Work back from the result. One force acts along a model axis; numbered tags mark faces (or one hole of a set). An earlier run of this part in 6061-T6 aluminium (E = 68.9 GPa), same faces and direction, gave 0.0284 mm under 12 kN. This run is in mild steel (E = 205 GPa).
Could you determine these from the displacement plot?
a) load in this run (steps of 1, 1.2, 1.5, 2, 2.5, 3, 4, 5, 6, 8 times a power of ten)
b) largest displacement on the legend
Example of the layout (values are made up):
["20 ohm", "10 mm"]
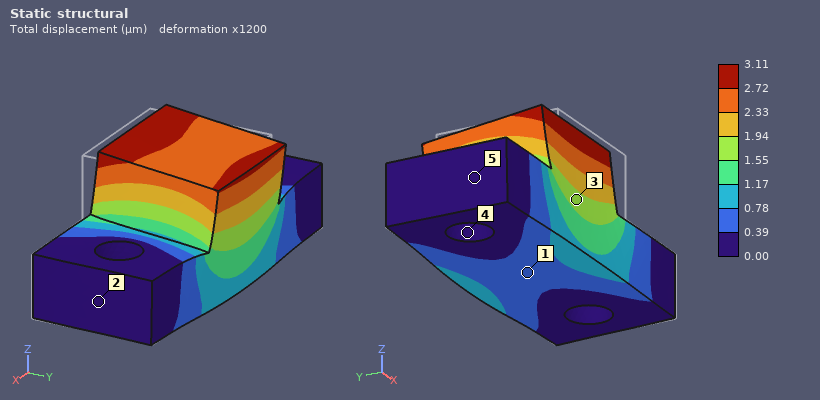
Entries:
["4 kN", "3.11 µm"]
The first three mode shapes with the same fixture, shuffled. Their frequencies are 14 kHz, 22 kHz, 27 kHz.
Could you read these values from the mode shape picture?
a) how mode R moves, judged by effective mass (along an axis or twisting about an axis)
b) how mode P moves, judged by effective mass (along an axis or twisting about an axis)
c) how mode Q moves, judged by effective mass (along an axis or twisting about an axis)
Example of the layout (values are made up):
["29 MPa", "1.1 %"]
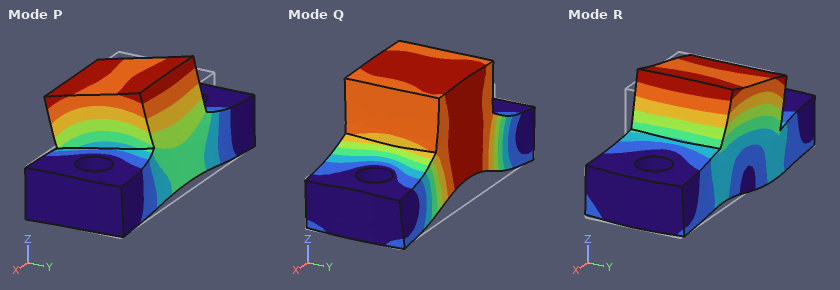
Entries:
["along X", "along Y", "along Z"]
